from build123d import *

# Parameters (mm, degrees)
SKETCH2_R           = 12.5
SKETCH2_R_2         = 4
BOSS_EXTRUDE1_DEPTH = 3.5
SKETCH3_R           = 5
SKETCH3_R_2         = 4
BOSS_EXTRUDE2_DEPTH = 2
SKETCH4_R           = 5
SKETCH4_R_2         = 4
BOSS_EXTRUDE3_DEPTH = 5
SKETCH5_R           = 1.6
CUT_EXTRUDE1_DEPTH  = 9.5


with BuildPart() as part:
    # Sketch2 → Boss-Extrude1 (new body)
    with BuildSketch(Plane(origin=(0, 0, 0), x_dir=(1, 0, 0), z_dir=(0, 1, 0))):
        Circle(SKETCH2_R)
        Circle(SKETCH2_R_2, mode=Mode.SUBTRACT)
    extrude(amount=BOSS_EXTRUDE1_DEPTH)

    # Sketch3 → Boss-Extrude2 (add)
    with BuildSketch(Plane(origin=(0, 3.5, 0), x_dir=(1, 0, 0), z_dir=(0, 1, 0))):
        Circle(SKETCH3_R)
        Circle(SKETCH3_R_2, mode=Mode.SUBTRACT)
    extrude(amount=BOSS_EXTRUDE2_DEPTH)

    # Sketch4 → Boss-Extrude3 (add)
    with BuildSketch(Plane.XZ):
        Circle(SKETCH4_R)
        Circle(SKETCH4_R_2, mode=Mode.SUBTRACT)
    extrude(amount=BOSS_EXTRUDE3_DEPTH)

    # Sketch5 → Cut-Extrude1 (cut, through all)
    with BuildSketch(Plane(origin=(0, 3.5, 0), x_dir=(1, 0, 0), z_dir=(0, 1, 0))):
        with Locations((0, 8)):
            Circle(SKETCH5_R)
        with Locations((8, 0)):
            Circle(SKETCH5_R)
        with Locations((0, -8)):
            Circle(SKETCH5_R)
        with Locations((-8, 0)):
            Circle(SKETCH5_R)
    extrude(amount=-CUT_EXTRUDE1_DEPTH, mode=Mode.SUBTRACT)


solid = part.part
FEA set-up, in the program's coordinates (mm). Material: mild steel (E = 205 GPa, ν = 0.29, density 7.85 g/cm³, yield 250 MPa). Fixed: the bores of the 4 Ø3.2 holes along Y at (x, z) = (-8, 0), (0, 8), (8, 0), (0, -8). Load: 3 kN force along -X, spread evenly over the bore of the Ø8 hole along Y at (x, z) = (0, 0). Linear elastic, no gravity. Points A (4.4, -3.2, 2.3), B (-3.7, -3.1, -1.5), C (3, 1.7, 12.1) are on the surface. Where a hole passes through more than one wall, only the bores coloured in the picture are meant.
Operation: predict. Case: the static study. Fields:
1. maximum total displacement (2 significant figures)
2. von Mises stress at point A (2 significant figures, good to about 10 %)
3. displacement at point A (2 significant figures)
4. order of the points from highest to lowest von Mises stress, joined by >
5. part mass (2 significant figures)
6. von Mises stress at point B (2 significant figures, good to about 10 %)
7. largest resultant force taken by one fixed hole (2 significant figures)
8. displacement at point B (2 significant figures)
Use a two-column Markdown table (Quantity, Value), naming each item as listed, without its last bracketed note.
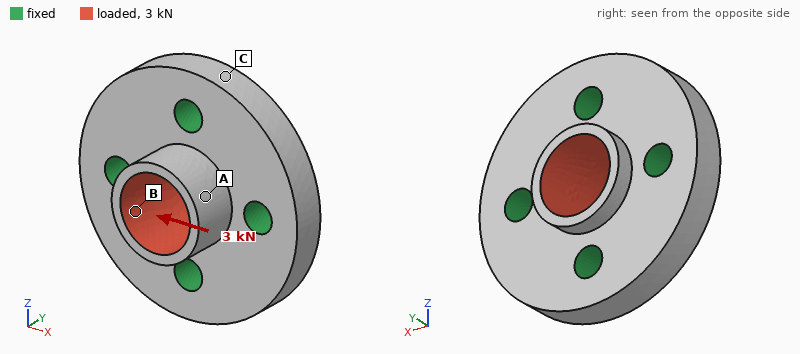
| Quantity | Value |
|---|---|
| maximum total displacement | 6.6 µm |
| von Mises stress at point A | 43 MPa |
| displacement at point A | 4.9 µm |
| order of the points from highest to lowest von Mises stress, joined by > | B > A > C |
| part mass | 13 g |
| von Mises stress at point B | 66 MPa |
| largest resultant force taken by one fixed hole | 890 N |
| displacement at point B | 4.8 µm |
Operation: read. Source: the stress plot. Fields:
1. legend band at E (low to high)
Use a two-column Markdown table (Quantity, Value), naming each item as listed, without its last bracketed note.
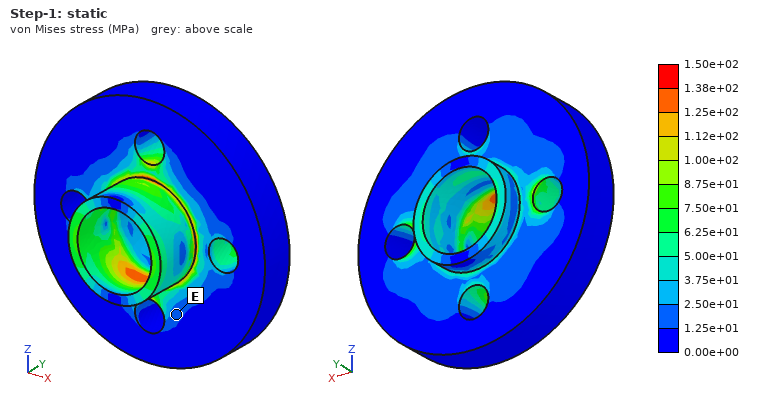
| Quantity | Value |
|---|---|
| legend band at E | 1.25e+01 to 2.50e+01 MPa |
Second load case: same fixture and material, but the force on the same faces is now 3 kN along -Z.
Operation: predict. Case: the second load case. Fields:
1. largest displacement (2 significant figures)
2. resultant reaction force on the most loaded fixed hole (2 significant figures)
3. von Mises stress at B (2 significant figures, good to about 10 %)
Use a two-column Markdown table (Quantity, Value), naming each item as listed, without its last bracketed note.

| Quantity | Value |
|---|---|
| largest displacement | 6.6 µm |
| resultant reaction force on the most loaded fixed hole | 890 N |
| von Mises stress at B | 84 MPa |
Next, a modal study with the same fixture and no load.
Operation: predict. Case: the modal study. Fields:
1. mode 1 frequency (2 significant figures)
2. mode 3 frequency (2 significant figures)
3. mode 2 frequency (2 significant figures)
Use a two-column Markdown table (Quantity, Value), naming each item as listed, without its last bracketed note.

| Quantity | Value |
|---|---|
| mode 1 frequency | 63 kHz |
| mode 3 frequency | 69 kHz |
| mode 2 frequency | 67 kHz |
